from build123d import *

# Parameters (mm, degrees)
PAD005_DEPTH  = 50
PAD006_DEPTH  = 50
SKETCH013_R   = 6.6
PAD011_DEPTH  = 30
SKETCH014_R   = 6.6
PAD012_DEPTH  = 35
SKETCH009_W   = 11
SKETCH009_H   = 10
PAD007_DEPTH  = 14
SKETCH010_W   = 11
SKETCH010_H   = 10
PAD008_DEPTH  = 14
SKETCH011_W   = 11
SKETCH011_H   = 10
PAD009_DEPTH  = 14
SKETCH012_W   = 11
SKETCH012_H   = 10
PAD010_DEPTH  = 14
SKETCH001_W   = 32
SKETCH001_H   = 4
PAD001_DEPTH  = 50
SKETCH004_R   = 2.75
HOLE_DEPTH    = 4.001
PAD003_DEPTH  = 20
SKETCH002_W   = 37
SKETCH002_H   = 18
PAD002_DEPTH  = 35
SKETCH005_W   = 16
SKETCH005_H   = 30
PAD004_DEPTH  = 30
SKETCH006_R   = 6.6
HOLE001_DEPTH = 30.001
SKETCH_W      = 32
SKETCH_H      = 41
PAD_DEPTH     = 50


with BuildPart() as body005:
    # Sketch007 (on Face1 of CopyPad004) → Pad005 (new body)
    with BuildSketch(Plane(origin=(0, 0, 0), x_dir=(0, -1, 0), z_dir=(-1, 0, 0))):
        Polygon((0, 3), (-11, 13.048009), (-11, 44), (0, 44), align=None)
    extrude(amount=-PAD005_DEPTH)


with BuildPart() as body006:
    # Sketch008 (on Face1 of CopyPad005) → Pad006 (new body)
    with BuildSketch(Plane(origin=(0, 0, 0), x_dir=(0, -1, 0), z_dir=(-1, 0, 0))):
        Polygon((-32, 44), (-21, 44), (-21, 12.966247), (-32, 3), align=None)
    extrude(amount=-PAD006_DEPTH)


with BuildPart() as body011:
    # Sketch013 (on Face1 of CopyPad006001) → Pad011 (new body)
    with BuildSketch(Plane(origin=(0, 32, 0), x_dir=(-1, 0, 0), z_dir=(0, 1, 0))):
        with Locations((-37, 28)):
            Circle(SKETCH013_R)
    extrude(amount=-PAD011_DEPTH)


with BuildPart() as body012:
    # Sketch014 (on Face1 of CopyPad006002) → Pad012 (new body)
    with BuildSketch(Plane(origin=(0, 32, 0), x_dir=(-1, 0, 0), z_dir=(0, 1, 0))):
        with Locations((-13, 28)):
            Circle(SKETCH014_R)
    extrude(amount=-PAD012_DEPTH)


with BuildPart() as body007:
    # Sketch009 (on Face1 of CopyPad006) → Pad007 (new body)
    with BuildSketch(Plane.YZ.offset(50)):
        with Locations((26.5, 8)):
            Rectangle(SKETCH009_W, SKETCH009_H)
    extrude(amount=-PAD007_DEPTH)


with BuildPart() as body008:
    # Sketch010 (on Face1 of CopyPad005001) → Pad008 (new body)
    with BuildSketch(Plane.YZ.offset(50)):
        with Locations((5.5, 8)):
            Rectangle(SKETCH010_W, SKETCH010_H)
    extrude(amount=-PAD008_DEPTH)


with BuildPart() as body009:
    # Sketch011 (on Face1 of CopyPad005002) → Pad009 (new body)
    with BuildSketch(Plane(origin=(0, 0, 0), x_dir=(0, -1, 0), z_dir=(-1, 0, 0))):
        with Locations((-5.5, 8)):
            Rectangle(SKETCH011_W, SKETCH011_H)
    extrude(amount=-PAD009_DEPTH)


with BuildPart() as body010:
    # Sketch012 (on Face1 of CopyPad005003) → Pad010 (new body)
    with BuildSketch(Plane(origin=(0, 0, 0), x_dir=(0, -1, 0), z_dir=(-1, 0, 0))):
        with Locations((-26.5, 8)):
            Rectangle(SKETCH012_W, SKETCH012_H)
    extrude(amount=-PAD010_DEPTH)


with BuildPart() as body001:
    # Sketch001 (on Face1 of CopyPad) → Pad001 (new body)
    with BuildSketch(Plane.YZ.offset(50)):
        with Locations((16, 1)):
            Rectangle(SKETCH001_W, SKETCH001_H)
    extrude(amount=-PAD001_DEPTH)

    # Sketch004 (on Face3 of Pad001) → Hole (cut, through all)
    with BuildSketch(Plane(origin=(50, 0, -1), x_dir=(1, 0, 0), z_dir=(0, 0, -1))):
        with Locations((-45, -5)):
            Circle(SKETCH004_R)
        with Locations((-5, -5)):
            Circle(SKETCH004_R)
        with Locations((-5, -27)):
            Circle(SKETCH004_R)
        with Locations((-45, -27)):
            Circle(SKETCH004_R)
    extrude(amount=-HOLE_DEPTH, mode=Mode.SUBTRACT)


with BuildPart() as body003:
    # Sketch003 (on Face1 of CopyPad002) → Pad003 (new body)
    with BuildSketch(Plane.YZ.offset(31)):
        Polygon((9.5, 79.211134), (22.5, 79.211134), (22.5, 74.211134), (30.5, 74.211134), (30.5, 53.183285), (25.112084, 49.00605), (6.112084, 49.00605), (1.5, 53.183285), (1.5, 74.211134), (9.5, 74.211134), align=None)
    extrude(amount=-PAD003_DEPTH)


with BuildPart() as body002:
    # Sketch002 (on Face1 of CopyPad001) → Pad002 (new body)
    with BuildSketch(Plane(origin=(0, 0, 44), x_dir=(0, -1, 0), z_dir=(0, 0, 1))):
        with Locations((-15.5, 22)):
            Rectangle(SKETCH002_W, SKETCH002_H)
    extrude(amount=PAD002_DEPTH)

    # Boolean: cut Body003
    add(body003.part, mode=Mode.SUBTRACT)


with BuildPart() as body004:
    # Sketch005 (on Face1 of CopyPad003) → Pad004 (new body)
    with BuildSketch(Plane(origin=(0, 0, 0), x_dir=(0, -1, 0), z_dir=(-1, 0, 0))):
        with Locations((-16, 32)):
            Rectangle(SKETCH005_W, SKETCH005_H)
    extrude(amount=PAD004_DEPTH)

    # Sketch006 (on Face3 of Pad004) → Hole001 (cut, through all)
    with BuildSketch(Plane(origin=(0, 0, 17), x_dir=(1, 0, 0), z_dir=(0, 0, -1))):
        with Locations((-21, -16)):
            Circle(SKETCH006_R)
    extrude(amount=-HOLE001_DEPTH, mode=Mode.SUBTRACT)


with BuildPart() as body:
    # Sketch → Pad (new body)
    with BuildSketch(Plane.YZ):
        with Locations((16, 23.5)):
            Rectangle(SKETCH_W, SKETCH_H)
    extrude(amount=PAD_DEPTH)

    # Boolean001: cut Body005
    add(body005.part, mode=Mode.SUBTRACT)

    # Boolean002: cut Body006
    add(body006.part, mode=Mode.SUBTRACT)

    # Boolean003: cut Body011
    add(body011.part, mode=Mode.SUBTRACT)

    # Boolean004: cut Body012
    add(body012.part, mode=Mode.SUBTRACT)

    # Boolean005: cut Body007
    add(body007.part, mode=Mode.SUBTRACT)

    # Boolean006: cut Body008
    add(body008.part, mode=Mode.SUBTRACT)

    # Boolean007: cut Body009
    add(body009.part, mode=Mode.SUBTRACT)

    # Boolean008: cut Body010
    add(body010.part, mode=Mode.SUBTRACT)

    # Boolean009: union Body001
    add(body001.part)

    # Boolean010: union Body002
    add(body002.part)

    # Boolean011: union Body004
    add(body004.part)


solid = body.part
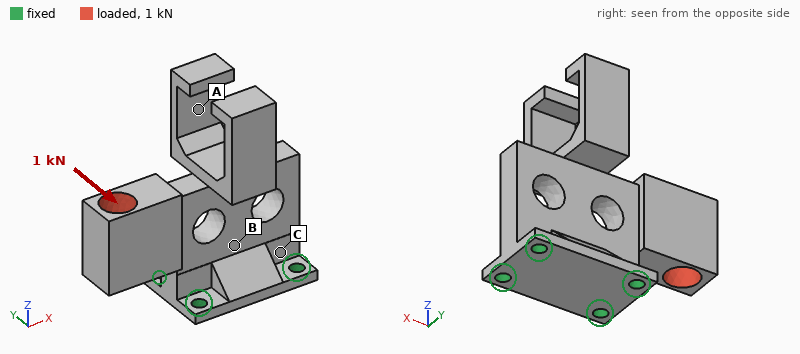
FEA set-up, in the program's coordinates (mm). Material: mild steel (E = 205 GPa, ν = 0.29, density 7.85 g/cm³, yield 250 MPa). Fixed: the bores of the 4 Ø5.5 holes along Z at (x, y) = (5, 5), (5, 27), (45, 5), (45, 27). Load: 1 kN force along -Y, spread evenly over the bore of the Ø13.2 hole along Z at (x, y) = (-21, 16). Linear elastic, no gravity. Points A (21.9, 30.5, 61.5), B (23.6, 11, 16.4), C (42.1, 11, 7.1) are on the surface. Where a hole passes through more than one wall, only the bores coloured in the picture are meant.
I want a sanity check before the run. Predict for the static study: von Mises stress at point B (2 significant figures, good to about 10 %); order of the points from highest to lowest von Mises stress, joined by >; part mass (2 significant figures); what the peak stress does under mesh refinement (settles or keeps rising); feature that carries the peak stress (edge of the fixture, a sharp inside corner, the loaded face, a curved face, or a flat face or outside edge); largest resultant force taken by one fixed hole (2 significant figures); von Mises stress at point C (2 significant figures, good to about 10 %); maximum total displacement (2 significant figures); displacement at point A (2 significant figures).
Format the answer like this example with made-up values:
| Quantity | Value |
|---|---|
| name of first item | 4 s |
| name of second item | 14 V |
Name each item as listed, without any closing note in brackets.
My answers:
| Quantity | Value |
|---|---|
| von Mises stress at point B | 30 MPa |
| order of the points from highest to lowest von Mises stress, joined by > | B > C > A |
| part mass | 360 g |
| what the peak stress does under mesh refinement | keeps rising |
| feature that carries the peak stress | a sharp inside corner |
| largest resultant force taken by one fixed hole | 1.5 kN |
| von Mises stress at point C | 16 MPa |
| maximum total displacement | 0.12 mm |
| displacement at point A | 0.038 mm |
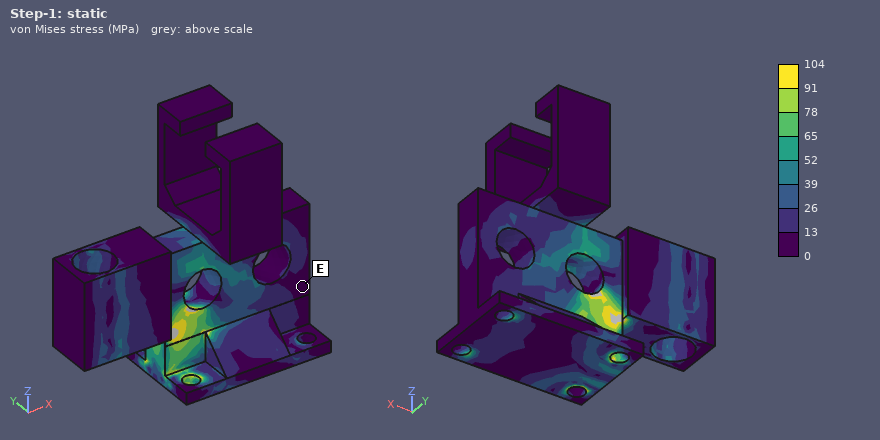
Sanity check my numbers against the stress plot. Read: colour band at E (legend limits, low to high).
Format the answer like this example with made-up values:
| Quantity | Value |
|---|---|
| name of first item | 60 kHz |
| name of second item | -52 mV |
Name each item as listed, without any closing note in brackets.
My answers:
| Quantity | Value |
|---|---|
| colour band at E | 0 to 13 MPa |
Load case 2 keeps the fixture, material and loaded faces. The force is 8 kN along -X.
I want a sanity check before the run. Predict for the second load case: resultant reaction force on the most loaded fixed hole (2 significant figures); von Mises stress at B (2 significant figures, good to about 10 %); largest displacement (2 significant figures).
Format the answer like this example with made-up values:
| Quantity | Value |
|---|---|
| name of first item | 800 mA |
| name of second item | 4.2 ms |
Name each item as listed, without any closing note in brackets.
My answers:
| Quantity | Value |
|---|---|
| resultant reaction force on the most loaded fixed hole | 4.0 kN |
| von Mises stress at B | 32 MPa |
| largest displacement | 74 µm |
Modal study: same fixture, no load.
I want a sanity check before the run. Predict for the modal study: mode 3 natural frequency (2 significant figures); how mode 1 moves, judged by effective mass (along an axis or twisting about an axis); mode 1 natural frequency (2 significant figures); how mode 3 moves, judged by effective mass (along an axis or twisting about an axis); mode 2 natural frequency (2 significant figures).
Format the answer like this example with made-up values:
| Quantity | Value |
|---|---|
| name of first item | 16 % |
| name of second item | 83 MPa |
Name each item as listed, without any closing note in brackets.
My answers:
| Quantity | Value |
|---|---|
| mode 3 natural frequency | 2400 Hz |
| how mode 1 moves, judged by effective mass | along Y |
| mode 1 natural frequency | 1200 Hz |
| how mode 3 moves, judged by effective mass | along Y |
| mode 2 natural frequency | 2000 Hz |
